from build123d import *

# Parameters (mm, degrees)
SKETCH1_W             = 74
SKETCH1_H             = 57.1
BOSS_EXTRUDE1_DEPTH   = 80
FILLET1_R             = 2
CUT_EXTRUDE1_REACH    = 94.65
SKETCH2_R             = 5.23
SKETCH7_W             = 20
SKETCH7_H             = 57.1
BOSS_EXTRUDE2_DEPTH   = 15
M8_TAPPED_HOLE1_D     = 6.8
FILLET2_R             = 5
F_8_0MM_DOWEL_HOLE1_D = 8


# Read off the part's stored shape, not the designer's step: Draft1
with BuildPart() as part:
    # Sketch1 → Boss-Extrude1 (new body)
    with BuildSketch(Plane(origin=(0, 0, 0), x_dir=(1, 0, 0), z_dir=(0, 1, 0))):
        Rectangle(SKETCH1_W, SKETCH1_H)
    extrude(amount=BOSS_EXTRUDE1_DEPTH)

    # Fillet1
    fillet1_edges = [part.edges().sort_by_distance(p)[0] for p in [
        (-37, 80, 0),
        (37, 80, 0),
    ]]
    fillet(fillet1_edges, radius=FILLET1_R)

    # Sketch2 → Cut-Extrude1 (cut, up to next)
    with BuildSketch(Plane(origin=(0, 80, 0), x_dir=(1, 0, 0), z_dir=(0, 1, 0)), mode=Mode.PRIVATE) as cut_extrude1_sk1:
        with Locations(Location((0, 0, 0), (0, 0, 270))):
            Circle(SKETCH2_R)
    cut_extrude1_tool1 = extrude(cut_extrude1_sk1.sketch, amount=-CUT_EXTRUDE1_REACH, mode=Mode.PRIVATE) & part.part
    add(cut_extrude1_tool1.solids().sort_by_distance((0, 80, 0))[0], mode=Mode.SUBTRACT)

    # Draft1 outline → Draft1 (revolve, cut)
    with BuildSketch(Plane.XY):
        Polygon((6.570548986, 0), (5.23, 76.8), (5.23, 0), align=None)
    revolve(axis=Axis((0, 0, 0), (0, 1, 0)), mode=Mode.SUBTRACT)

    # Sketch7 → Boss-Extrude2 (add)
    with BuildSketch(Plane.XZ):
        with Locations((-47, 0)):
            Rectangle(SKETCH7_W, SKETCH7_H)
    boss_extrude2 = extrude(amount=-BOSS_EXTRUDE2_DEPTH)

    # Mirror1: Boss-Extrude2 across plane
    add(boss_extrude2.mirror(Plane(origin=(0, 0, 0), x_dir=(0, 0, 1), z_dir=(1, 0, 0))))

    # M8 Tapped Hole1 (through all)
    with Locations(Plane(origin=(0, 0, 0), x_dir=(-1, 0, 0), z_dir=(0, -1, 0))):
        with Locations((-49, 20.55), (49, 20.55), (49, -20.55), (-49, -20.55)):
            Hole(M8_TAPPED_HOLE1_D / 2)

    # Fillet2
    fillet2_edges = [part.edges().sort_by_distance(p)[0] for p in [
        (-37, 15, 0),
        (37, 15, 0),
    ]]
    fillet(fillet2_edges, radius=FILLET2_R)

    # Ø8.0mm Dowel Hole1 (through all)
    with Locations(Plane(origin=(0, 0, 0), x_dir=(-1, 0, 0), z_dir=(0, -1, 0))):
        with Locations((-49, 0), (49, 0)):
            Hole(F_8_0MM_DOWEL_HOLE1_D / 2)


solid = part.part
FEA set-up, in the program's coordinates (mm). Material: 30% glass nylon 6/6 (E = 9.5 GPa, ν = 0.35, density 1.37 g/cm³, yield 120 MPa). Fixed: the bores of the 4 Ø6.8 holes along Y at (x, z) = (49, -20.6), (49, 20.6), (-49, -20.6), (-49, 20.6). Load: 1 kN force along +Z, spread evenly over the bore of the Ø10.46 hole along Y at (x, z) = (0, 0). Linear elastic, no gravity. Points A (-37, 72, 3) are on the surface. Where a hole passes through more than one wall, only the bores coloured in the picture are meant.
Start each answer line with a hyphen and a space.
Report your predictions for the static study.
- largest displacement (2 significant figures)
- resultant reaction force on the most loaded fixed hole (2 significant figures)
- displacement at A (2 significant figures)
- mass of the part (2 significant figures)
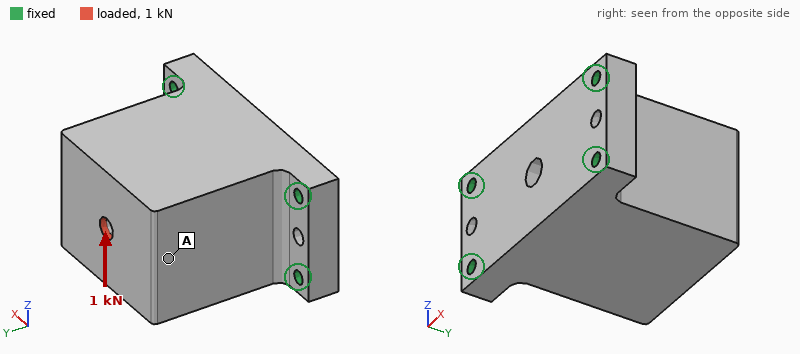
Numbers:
- 93 µm
- 930 N
- 74 µm
- 490 g
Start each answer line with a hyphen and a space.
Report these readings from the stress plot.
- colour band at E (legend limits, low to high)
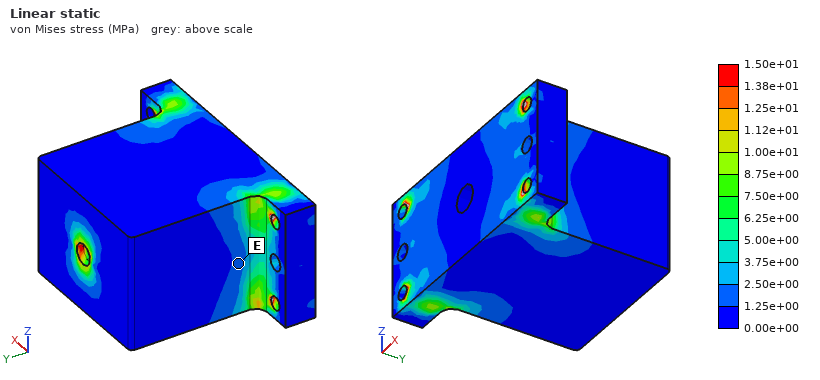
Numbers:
- 1.25e+00 to 2.50e+00 MPa
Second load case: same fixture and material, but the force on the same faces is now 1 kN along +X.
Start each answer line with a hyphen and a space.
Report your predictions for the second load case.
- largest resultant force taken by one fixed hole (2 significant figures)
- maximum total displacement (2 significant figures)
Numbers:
- 480 N
- 31 µm
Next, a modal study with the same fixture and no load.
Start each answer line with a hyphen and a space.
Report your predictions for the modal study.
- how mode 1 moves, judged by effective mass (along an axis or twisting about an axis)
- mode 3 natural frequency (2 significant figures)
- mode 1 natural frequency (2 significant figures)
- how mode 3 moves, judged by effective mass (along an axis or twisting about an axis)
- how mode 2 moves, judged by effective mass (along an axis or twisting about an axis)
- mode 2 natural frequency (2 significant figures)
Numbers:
- along Z
- 2900 Hz
- 1400 Hz
- along Y
- along X
- 2600 Hz
